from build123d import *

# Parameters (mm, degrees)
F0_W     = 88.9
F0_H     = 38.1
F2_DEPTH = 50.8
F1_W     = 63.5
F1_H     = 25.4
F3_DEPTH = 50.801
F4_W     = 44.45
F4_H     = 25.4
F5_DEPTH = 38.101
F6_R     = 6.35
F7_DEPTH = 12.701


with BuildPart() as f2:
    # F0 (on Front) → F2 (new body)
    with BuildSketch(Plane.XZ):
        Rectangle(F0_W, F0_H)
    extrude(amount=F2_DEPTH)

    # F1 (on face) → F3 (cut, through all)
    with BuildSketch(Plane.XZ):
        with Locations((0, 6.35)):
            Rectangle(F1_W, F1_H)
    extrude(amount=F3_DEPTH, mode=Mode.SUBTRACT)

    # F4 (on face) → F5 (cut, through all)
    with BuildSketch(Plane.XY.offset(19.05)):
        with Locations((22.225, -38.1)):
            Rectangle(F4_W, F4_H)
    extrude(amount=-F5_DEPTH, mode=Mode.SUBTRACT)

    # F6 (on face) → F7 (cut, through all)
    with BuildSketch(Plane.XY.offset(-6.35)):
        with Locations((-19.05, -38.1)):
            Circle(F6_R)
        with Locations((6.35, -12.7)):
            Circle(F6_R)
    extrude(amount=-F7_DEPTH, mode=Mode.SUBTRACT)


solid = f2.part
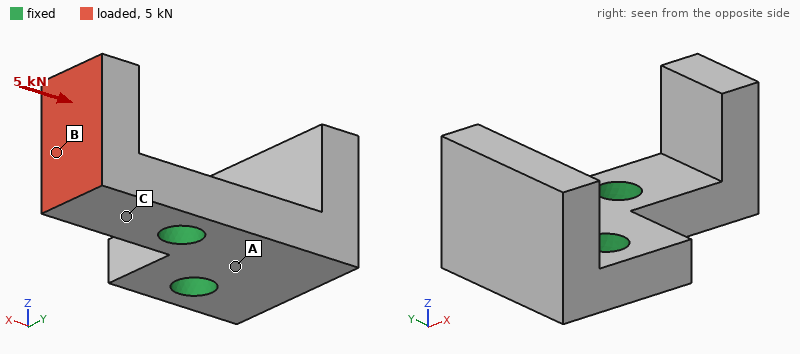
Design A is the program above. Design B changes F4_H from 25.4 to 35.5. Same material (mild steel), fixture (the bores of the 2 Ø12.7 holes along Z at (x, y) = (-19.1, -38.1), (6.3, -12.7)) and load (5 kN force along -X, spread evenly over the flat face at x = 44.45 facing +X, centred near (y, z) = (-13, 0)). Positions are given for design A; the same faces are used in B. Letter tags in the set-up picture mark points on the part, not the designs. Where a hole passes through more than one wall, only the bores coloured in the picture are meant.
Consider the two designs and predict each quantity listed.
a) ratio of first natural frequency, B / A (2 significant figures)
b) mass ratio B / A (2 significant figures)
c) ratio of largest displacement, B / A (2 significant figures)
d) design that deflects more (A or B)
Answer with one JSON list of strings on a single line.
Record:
["1.0", "0.93", "1.2", "B"]
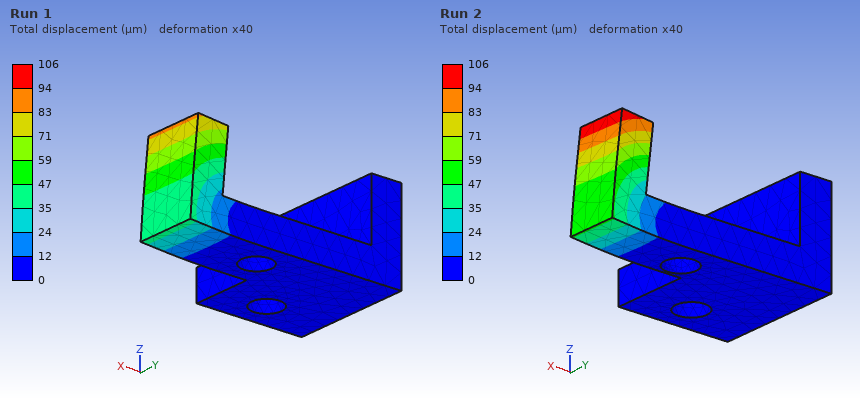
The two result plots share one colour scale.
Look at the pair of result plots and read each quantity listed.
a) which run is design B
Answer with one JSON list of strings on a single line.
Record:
["Run 2"]
